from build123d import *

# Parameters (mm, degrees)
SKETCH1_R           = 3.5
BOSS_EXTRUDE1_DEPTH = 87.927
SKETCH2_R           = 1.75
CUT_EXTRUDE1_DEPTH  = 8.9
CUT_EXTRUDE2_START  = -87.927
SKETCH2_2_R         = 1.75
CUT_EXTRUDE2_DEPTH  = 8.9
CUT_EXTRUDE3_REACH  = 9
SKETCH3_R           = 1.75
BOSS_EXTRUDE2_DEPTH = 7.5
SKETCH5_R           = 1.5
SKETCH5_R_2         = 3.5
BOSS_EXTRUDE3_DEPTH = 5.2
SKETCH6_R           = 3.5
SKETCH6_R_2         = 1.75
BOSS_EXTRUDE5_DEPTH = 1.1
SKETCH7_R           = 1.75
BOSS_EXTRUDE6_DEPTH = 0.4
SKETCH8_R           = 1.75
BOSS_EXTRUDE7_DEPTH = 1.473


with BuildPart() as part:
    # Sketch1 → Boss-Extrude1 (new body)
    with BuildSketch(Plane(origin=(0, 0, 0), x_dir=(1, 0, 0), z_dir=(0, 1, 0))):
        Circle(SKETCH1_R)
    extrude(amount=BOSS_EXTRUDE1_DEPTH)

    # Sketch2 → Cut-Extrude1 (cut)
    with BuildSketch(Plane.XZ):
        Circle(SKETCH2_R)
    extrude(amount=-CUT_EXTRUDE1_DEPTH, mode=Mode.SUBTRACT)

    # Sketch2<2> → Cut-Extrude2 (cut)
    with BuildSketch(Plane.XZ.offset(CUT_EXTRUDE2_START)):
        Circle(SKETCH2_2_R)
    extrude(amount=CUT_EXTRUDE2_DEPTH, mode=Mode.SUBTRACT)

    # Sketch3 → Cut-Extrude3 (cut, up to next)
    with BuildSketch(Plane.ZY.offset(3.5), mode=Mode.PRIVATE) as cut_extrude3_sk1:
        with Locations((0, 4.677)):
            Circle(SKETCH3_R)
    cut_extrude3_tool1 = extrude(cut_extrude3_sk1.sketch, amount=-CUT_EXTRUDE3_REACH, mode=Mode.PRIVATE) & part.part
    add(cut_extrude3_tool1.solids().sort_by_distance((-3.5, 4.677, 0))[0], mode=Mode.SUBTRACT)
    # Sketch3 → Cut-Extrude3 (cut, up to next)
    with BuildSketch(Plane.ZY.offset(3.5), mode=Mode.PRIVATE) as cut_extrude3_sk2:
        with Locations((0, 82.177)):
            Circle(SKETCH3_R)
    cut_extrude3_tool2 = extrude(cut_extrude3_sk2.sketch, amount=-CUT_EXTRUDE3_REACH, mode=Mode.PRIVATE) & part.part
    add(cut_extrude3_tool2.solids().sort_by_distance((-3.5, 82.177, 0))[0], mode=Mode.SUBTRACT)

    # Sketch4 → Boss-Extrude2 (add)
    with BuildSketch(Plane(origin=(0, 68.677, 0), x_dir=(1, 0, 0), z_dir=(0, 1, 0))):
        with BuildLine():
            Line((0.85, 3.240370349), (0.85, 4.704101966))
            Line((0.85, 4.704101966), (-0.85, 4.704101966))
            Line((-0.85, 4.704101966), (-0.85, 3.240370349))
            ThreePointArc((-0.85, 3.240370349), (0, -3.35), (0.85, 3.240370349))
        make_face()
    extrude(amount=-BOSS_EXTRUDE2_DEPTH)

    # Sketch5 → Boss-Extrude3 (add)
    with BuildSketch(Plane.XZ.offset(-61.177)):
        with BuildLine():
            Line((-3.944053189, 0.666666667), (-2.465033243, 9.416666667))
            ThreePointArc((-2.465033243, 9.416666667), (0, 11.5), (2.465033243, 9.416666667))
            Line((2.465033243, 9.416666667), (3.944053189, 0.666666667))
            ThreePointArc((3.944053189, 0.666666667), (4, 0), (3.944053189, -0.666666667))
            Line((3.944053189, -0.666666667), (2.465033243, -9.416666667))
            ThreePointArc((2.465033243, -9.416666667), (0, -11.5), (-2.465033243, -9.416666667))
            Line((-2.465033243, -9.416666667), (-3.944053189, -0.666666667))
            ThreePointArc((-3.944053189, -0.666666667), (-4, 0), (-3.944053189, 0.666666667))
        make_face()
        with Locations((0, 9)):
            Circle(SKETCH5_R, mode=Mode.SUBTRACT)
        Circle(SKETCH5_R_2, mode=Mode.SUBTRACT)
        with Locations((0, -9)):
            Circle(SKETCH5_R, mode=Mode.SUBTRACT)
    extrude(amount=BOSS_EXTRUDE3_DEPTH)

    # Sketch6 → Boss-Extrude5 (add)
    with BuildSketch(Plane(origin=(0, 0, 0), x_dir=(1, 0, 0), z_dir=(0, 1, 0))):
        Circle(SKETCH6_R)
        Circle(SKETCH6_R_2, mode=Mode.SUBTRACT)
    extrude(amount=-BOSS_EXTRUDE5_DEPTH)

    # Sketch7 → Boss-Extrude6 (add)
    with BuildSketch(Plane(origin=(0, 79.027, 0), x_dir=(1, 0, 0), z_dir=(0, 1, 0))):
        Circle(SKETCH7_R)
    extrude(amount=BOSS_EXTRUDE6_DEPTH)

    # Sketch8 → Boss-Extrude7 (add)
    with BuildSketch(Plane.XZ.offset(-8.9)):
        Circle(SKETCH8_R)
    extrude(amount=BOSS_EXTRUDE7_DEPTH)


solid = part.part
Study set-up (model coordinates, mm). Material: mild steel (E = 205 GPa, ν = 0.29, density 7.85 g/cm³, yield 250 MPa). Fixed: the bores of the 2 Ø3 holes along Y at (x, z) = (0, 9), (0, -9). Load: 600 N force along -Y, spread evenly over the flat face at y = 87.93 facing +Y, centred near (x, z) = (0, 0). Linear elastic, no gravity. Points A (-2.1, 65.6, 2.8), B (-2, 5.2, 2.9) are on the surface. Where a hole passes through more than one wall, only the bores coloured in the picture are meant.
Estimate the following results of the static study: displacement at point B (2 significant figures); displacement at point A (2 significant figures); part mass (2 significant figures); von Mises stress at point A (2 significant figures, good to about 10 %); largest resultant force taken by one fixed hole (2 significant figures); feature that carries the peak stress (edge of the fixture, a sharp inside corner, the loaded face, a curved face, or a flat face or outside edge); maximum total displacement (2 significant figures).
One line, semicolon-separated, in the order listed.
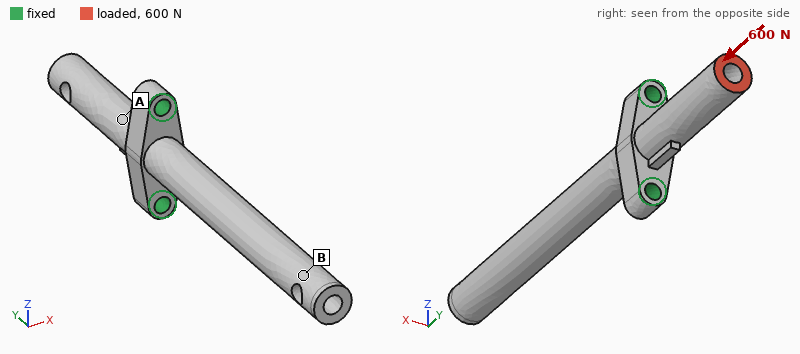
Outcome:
1.0 µm; 1.6 µm; 29 g; 17 MPa; 300 N; a curved face; 4.9 µm
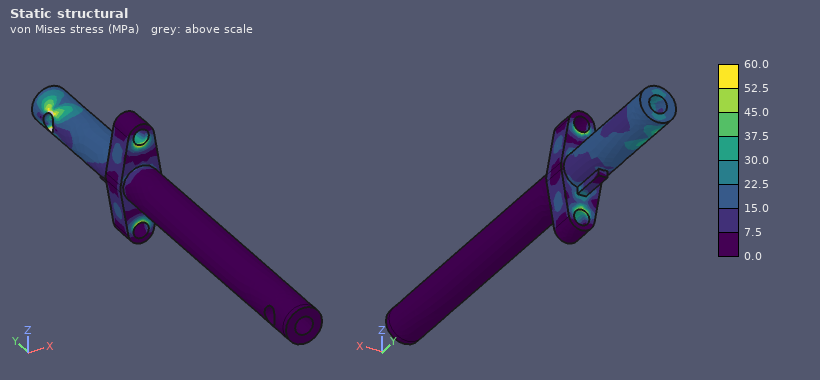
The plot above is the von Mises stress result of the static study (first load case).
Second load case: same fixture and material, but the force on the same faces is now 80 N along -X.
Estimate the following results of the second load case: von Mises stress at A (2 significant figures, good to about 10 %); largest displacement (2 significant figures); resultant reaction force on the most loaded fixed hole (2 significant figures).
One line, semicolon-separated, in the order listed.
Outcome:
32 MPa; 43 µm; 41 N
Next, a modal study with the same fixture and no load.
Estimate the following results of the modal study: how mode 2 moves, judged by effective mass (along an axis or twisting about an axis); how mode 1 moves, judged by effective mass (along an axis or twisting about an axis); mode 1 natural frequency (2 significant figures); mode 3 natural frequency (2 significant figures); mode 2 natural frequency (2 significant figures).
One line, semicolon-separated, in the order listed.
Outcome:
along Z; along X; 1300 Hz; 5200 Hz; 1500 Hz
